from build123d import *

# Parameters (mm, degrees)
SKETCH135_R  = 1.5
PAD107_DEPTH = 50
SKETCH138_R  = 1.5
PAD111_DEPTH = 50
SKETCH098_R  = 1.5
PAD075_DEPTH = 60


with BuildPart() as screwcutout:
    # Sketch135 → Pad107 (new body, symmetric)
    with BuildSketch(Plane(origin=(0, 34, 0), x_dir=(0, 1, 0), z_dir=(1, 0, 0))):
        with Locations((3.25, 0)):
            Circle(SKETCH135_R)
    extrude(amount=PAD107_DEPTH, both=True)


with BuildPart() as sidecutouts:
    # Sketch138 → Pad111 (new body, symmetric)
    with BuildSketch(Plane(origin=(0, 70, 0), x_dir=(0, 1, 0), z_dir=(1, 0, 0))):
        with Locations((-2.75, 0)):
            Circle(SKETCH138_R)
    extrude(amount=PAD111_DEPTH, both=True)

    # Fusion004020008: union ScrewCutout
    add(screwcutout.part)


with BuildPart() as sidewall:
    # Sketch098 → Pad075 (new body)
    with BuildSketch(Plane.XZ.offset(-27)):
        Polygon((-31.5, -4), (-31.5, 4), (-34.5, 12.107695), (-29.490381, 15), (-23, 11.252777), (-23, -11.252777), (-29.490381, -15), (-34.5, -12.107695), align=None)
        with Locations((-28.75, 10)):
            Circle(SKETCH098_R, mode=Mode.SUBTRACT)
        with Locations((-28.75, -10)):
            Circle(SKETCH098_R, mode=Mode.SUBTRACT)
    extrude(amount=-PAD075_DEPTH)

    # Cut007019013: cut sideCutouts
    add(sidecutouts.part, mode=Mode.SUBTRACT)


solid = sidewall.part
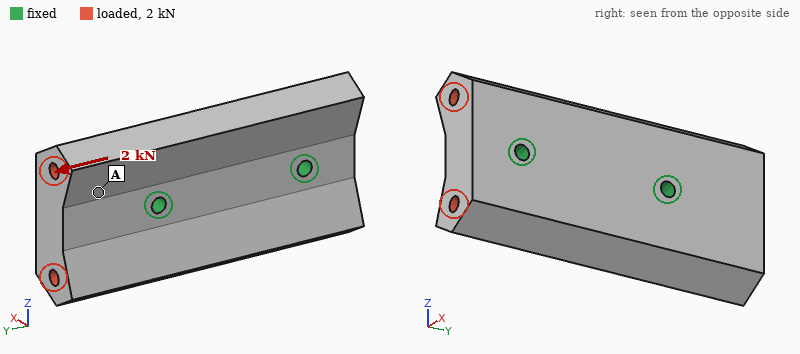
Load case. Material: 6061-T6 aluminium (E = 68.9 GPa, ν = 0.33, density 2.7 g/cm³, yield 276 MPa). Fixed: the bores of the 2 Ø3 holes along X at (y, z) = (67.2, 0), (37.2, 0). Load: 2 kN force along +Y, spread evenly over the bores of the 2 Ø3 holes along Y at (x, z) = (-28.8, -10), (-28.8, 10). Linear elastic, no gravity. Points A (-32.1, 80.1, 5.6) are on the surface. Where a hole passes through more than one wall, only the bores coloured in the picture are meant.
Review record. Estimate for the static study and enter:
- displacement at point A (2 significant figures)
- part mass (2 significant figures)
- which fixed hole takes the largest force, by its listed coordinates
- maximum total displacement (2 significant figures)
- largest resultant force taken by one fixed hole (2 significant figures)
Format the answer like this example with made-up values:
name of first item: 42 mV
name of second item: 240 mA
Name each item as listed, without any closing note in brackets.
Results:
displacement at point A: 1.8 µm
part mass: 39 g
which fixed hole takes the largest force, by its listed coordinates: (67.2, 0)
maximum total displacement: 2.5 µm
largest resultant force taken by one fixed hole: 1.1 kN
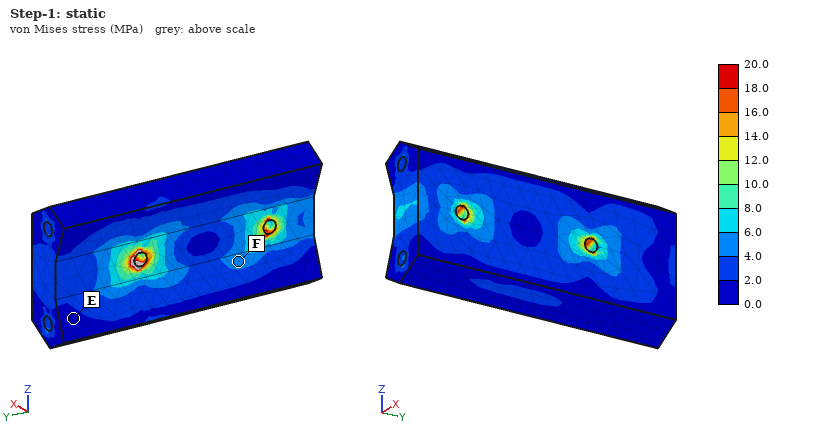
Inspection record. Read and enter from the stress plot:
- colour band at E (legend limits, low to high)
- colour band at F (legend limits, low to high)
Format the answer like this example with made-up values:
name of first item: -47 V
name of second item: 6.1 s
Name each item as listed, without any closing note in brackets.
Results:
colour band at E: 0.0 to 2.0 MPa
colour band at F: 4.0 to 6.0 MPa
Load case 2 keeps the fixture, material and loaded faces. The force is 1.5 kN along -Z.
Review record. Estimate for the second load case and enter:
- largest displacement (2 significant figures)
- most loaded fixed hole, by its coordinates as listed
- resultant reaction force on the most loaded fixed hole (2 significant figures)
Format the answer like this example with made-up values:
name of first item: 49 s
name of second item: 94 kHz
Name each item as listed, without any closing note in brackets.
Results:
largest displacement: 4.2 µm
most loaded fixed hole, by its coordinates as listed: (67.2, 0)
resultant reaction force on the most loaded fixed hole: 970 N
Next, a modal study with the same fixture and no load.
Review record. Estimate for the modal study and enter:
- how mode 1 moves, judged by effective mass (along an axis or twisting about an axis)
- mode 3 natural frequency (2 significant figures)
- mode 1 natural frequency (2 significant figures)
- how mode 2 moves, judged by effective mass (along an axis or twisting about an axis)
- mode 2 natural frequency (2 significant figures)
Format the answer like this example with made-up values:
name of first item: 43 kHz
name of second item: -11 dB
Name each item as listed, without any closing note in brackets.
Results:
how mode 1 moves, judged by effective mass: along X
mode 3 natural frequency: 18 kHz
mode 1 natural frequency: 13 kHz
how mode 2 moves, judged by effective mass: twisting about Y
mode 2 natural frequency: 14 kHz
